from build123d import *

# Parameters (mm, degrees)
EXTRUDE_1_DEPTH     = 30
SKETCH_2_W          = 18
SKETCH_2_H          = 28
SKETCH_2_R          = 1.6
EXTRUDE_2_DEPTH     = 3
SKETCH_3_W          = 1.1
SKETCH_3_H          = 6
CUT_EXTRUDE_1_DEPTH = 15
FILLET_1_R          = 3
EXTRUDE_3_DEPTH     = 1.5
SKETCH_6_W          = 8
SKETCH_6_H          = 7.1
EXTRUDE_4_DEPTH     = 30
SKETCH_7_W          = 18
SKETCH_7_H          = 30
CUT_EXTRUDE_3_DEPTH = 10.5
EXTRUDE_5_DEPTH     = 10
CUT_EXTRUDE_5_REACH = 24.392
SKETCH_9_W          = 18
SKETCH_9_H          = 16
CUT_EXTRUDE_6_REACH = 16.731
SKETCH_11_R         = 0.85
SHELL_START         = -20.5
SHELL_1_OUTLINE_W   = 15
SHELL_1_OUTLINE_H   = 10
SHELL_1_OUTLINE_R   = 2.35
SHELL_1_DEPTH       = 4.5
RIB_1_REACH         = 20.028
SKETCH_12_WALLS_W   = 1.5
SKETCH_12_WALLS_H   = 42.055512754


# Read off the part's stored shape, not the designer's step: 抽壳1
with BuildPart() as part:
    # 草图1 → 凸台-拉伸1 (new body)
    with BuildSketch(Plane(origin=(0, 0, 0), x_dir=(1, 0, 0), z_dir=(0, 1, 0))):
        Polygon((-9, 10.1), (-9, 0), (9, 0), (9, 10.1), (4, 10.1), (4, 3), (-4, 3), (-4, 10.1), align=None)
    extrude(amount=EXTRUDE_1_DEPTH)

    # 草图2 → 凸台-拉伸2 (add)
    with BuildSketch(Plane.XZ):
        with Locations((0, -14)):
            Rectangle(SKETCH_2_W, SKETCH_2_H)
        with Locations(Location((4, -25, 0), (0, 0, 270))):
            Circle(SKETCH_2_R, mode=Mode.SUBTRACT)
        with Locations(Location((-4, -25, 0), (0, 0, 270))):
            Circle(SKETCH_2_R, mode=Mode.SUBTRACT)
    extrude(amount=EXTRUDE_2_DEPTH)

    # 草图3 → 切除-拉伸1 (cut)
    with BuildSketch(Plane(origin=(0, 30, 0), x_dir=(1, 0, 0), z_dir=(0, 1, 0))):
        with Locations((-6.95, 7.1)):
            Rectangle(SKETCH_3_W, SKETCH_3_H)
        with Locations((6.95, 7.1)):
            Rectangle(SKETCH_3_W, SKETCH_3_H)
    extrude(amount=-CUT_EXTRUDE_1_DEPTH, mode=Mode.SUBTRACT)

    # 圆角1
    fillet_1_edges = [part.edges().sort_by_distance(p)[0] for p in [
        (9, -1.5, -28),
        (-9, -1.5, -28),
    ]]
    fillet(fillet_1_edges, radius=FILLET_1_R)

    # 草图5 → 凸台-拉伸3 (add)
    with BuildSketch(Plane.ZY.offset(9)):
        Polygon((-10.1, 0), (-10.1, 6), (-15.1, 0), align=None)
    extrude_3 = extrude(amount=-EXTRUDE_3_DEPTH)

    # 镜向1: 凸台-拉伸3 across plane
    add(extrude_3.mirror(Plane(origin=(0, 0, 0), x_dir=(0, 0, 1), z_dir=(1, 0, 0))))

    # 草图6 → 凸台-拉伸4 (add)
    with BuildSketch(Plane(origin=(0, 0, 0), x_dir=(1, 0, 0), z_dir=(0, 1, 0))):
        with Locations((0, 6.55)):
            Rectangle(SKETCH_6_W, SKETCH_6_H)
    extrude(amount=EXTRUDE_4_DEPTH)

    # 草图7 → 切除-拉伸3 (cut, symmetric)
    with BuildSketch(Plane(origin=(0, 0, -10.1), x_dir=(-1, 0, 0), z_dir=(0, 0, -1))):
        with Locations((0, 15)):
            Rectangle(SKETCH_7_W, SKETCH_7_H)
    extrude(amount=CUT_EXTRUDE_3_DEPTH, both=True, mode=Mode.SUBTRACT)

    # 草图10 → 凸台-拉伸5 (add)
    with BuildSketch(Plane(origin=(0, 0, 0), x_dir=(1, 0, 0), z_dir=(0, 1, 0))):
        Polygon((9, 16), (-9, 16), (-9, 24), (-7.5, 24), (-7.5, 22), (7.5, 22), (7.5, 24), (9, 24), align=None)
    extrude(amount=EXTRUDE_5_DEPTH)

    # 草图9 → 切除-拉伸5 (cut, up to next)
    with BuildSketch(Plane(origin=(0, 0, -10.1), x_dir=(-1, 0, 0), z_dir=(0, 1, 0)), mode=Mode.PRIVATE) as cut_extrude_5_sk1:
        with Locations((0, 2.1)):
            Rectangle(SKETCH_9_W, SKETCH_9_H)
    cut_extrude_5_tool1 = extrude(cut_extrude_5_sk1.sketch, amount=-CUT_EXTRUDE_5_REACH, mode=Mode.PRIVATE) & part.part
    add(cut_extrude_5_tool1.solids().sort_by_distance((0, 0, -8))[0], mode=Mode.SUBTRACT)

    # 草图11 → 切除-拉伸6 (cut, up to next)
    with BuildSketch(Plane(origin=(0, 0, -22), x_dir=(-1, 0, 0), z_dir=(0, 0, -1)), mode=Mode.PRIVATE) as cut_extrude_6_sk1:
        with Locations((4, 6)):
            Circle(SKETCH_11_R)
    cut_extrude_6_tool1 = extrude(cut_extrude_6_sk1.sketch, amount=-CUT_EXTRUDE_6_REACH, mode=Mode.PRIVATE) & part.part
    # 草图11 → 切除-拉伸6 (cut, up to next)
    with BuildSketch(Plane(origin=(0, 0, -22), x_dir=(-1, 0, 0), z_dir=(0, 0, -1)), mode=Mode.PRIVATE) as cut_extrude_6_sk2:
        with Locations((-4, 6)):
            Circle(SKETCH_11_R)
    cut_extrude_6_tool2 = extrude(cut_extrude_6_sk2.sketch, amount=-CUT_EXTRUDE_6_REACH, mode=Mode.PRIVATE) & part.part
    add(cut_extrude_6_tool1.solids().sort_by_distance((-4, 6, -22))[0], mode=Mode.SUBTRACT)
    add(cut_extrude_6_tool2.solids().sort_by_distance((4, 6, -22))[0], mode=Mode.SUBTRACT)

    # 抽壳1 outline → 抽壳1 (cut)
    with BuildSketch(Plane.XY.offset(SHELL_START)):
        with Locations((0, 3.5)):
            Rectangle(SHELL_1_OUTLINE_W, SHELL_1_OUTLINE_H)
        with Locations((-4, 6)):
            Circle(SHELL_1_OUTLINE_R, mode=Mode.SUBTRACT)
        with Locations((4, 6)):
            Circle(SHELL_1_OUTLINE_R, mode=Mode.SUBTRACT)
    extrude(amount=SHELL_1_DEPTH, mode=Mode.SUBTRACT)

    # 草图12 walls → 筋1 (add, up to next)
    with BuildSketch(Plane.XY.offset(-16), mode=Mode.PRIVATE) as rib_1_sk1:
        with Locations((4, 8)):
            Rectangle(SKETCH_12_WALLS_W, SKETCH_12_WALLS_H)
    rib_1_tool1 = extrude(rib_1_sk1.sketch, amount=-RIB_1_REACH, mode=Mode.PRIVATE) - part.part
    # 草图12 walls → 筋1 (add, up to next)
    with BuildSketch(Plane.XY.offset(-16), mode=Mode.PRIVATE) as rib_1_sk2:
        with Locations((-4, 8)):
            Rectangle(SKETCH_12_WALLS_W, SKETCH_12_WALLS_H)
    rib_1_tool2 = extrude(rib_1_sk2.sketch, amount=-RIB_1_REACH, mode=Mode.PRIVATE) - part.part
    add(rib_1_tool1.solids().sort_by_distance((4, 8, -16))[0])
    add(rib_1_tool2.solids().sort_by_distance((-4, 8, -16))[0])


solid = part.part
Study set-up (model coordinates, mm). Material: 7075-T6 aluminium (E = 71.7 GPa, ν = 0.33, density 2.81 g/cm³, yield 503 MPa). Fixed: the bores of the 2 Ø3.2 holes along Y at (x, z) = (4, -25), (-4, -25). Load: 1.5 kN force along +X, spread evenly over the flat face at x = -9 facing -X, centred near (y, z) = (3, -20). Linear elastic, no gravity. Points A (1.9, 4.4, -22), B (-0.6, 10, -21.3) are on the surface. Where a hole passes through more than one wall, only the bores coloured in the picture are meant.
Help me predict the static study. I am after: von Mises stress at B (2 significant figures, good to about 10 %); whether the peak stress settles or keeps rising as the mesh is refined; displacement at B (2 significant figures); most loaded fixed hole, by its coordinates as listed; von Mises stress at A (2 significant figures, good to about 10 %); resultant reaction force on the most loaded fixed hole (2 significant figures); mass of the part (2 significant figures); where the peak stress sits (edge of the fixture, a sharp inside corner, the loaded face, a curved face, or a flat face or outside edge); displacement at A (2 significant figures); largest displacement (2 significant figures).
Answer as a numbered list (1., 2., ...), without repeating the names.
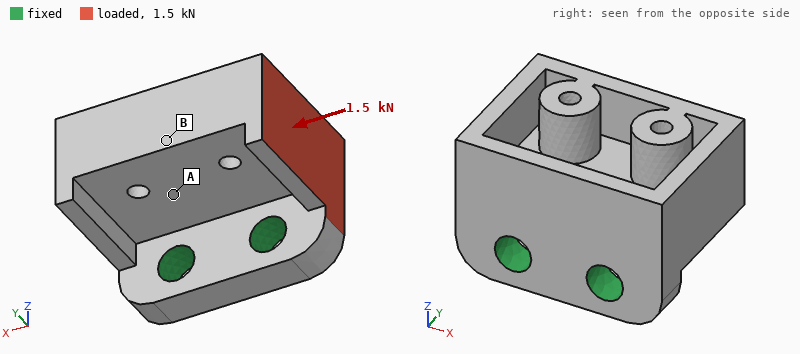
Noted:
1. 21 MPa
2. keeps rising
3. 30 µm
4. (-4, -25)
5. 58 MPa
6. 1.1 kN
7. 3.3 g
8. edge of the fixture
9. 17 µm
10. 55 µm
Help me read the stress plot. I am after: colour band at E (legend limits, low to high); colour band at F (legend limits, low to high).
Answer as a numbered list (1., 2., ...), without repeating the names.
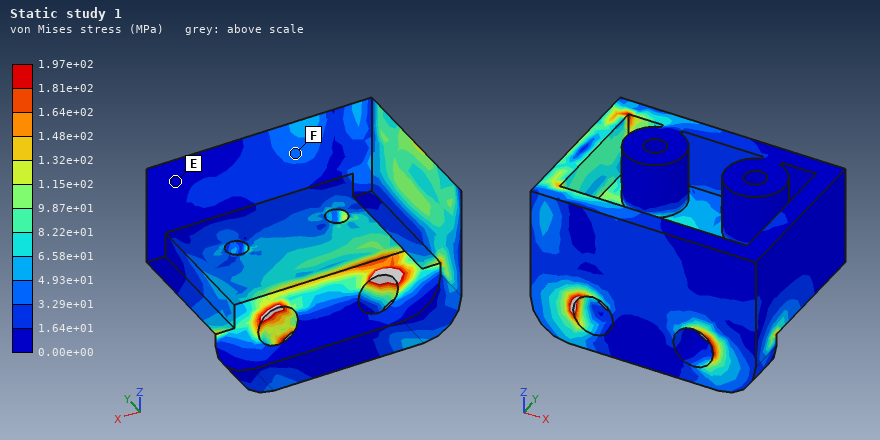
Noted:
1. 0.00e+00 to 1.64e+01 MPa
2. 3.29e+01 to 4.93e+01 MPa
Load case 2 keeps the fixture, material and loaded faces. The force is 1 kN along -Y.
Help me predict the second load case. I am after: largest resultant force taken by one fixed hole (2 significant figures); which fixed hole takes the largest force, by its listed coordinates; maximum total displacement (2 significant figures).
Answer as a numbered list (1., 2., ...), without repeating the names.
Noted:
1. 1.3 kN
2. (-4, -25)
3. 0.12 mm
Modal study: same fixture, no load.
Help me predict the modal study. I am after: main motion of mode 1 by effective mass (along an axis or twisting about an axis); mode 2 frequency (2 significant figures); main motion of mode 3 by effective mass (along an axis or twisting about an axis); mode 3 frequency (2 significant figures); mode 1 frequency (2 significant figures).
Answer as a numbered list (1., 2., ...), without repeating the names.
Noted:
1. along Z
2. 16 kHz
3. along X
4. 22 kHz
5. 9800 Hz
